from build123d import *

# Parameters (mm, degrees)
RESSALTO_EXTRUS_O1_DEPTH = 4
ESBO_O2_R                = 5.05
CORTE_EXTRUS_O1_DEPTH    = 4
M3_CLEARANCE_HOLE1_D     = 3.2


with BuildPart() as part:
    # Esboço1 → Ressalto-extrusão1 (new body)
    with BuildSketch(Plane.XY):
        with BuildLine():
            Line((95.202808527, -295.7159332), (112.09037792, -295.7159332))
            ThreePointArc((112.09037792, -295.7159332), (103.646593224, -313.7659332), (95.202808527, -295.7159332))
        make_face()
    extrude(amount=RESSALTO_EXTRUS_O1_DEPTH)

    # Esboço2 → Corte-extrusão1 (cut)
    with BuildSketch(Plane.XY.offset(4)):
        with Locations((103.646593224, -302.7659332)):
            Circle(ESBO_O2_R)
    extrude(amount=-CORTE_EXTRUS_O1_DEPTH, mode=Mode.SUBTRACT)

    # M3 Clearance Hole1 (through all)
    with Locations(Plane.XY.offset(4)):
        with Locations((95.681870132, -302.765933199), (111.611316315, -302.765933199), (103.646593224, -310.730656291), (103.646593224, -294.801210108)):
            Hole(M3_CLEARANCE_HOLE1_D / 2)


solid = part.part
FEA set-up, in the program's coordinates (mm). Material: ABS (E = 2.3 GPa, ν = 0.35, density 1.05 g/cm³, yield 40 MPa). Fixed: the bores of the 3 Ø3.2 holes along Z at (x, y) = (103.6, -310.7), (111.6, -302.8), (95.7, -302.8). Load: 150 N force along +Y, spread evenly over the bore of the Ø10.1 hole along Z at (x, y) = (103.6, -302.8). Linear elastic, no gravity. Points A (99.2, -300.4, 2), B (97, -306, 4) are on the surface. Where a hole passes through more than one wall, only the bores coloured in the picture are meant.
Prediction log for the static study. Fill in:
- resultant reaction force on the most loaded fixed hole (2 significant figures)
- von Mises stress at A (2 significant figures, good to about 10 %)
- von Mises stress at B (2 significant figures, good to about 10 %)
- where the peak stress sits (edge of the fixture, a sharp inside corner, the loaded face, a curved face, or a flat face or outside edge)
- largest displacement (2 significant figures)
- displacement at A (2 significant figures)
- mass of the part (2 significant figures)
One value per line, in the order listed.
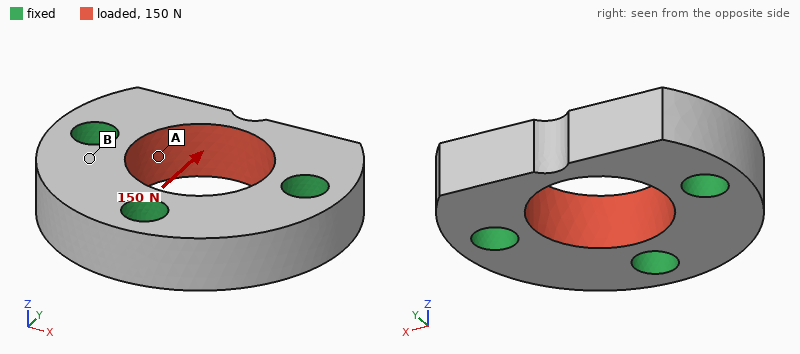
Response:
58 N
5.8 MPa
0.94 MPa
a curved face
27 µm
7.5 µm
0.96 g
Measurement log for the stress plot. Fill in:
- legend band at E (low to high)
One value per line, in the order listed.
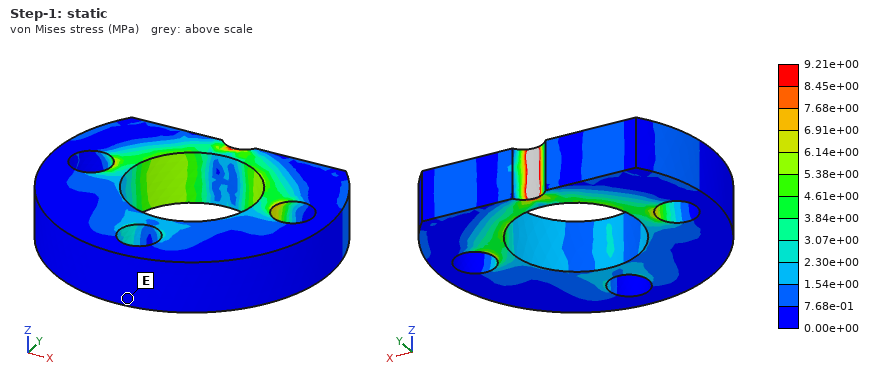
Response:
0.00e+00 to 7.68e-01 MPa
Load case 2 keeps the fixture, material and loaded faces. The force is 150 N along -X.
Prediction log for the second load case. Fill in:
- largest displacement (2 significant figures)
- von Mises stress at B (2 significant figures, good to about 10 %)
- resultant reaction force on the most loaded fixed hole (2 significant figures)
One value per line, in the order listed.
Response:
15 µm
1.0 MPa
58 N
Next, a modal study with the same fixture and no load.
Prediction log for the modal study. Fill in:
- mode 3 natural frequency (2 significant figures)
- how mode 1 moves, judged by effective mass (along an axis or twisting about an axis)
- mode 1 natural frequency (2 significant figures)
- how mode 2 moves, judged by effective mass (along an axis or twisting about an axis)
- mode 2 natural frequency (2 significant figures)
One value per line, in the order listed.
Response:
22 kHz
along Z
14 kHz
along X
21 kHz
